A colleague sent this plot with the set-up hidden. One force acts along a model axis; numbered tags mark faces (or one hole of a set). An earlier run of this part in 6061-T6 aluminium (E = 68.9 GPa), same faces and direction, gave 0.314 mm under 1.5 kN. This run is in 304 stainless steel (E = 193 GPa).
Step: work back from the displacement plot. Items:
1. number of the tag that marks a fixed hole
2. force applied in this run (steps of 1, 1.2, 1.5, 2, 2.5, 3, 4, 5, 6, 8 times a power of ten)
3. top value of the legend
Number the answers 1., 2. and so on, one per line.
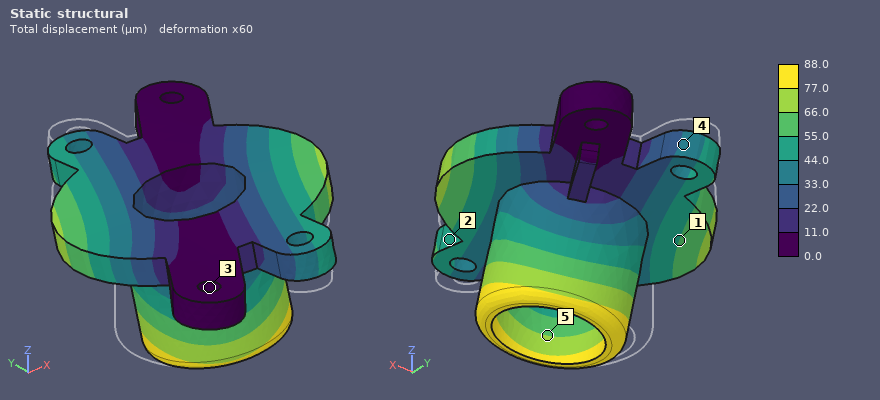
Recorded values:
1. 3
2. 1.2 kN
3. 88.0 µm
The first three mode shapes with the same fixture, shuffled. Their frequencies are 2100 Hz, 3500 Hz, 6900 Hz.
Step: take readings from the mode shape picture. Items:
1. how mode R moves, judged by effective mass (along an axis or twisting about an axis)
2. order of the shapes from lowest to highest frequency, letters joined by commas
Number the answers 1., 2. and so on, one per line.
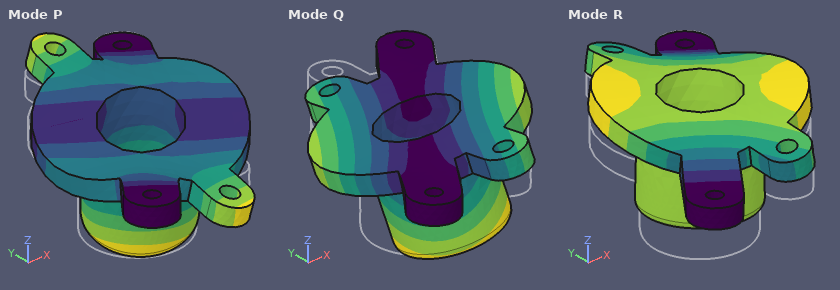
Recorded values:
1. along Z
2. Q, R, P
